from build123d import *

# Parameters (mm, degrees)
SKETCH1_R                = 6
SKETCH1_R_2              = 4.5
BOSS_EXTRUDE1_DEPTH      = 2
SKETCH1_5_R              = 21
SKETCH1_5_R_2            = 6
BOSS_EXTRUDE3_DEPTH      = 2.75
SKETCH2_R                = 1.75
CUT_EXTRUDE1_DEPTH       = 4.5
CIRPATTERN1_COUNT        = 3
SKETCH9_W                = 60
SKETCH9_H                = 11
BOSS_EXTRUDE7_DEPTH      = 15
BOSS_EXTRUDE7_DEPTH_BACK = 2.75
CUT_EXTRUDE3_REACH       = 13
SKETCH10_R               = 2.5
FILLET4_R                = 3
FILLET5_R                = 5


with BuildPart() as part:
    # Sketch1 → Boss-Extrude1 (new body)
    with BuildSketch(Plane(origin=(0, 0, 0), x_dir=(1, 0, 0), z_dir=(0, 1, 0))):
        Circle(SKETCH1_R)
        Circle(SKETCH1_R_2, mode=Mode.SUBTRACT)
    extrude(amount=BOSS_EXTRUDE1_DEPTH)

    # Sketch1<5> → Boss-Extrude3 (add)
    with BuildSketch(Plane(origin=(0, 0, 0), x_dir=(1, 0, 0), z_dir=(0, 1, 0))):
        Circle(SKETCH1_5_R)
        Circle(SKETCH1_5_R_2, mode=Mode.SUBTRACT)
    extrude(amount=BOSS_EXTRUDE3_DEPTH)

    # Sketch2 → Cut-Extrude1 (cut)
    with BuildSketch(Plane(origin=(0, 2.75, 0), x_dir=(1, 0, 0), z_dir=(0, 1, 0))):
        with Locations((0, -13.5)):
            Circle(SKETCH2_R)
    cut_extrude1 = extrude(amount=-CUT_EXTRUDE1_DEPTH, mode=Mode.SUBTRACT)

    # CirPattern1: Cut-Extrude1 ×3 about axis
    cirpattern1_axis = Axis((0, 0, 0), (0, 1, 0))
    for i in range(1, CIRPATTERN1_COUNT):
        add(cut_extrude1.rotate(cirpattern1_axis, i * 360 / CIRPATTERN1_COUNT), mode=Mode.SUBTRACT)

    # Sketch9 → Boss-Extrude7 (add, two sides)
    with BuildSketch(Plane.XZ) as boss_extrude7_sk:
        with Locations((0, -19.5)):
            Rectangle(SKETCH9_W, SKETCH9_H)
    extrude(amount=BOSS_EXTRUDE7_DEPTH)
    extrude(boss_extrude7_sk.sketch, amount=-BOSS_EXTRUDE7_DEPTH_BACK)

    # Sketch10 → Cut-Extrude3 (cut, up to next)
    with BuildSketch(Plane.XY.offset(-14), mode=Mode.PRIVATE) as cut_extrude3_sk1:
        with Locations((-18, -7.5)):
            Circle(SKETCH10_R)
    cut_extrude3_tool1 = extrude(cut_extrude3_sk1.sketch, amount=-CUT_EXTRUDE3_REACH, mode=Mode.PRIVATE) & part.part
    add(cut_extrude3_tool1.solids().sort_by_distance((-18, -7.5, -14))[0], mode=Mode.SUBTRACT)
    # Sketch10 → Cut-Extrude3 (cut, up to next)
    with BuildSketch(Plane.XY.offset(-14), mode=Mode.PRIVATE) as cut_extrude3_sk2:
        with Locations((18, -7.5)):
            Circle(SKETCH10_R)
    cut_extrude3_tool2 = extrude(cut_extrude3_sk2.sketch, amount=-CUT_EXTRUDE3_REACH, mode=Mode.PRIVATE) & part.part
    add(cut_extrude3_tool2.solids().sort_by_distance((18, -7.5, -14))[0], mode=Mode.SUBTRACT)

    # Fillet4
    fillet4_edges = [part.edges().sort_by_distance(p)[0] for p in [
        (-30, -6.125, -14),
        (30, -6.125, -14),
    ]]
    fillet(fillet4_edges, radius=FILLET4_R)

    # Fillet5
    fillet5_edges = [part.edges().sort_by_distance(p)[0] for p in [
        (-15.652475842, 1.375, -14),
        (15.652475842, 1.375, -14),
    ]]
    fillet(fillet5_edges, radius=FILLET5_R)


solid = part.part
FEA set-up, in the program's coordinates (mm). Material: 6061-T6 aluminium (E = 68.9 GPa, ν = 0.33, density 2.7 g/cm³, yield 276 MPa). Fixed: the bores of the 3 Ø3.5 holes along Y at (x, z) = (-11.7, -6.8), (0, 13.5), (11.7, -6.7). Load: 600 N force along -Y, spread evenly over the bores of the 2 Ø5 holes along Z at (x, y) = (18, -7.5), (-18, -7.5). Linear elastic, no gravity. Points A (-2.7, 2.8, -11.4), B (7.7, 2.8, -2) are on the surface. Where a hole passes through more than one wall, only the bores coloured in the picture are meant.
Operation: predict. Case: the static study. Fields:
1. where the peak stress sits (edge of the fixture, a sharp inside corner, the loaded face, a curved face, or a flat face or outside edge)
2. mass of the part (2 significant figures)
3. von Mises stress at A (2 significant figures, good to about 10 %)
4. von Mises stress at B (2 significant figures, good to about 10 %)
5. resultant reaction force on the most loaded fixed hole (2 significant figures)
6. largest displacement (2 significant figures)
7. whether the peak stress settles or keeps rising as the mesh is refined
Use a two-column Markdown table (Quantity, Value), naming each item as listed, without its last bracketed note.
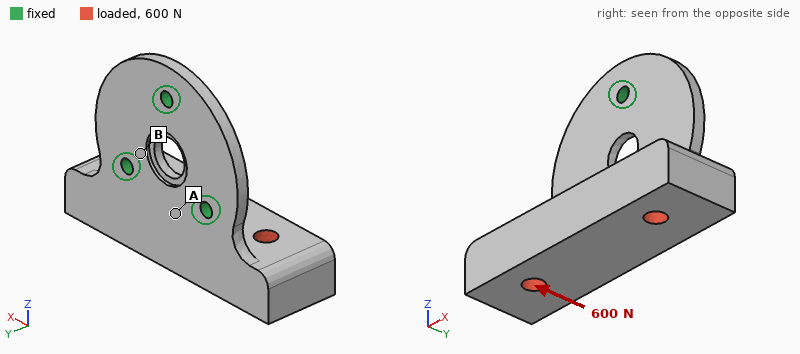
| Quantity | Value |
|---|---|
| where the peak stress sits | edge of the fixture |
| mass of the part | 39 g |
| von Mises stress at A | 63 MPa |
| von Mises stress at B | 21 MPa |
| resultant reaction force on the most loaded fixed hole | 320 N |
| largest displacement | 0.20 mm |
| whether the peak stress settles or keeps rising as the mesh is refined | keeps rising |
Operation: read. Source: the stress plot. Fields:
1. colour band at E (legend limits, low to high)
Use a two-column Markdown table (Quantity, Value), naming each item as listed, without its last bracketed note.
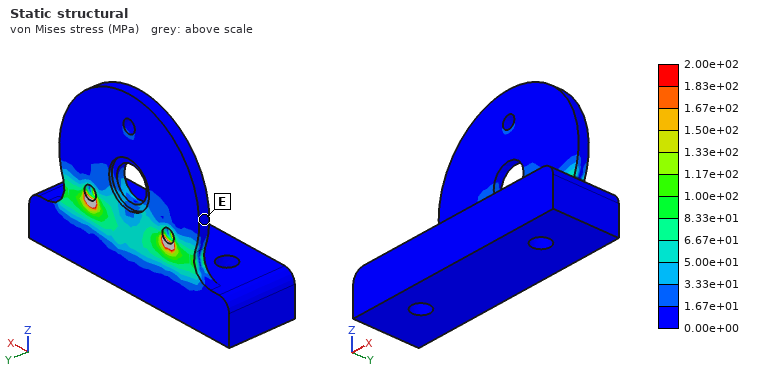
| Quantity | Value |
|---|---|
| colour band at E | 0.00e+00 to 1.67e+01 MPa |
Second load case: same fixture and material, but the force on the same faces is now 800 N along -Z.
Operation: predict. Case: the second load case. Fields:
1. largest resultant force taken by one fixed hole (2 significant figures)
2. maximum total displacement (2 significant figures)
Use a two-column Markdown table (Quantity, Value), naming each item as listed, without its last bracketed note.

| Quantity | Value |
|---|---|
| largest resultant force taken by one fixed hole | 370 N |
| maximum total displacement | 0.27 mm |
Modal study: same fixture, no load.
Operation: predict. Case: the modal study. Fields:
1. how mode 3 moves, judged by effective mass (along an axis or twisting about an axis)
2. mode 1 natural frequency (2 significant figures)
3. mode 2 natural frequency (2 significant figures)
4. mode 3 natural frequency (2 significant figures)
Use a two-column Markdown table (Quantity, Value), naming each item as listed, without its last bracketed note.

| Quantity | Value |
|---|---|
| how mode 3 moves, judged by effective mass | along X |
| mode 1 natural frequency | 1700 Hz |
| mode 2 natural frequency | 4100 Hz |
| mode 3 natural frequency | 8800 Hz |
